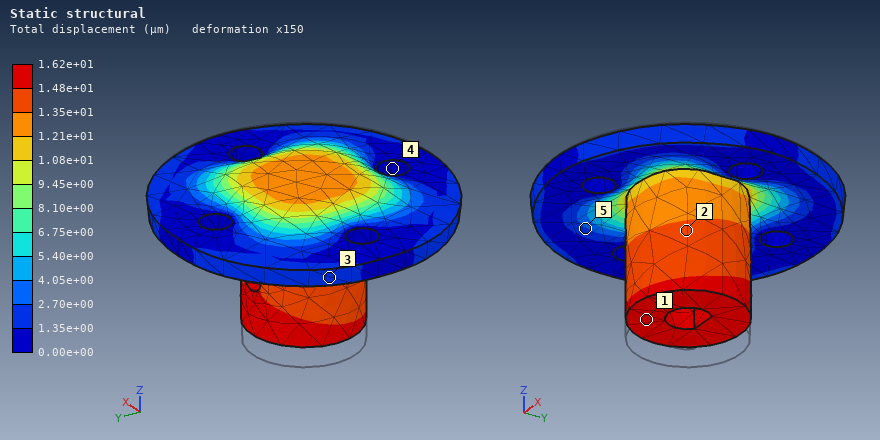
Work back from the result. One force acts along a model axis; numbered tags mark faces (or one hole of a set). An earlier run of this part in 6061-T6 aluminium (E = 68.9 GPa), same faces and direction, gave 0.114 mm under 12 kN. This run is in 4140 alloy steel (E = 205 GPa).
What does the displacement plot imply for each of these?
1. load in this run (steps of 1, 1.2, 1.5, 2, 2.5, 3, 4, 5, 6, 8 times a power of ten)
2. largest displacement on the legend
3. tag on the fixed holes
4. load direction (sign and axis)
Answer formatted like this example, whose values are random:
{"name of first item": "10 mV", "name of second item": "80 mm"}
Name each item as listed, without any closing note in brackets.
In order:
{"load in this run": "5 kN", "largest displacement on the legend": "1.62e+01 µm", "tag on the fixed holes": "4", "load direction": "+Z"}
